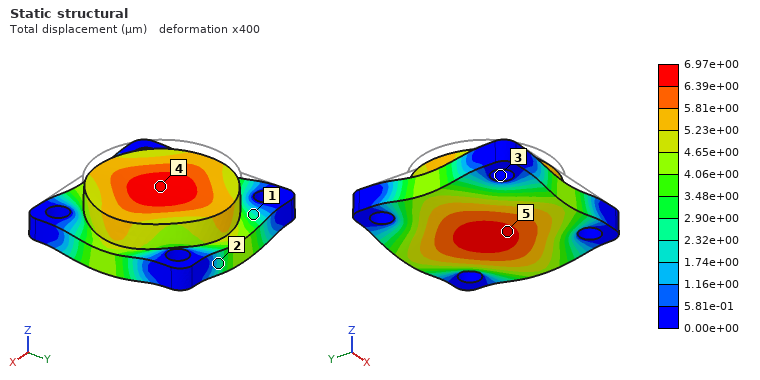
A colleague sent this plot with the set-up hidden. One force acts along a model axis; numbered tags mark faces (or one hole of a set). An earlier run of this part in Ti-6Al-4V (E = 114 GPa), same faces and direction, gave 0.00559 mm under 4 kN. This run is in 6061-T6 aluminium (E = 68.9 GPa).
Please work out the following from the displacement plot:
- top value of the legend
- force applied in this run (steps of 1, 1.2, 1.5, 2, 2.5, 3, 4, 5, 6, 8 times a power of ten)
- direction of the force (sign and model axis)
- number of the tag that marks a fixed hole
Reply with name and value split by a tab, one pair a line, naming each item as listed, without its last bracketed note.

top value of the legend	6.97e+00 µm
force applied in this run	3 kN
direction of the force	-Z
number of the tag that marks a fixed hole	3
